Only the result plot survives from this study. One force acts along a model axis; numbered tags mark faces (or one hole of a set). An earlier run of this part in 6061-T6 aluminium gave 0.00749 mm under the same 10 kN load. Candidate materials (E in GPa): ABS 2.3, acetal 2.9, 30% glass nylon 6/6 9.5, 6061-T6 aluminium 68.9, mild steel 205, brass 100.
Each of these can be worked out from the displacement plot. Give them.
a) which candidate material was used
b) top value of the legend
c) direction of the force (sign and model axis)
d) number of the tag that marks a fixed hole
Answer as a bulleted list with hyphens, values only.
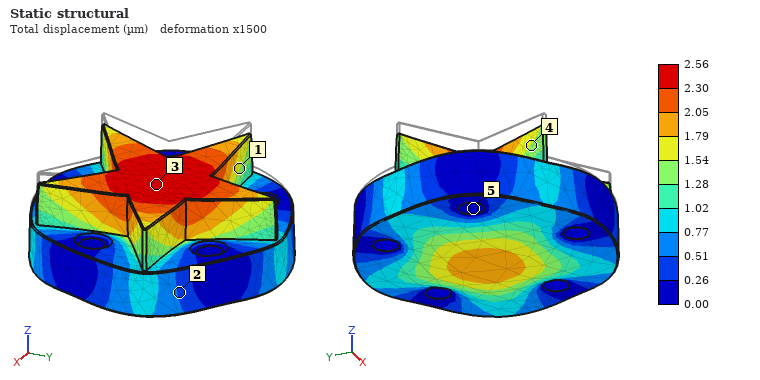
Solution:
- mild steel
- 2.56 µm
- -Z
- 5
